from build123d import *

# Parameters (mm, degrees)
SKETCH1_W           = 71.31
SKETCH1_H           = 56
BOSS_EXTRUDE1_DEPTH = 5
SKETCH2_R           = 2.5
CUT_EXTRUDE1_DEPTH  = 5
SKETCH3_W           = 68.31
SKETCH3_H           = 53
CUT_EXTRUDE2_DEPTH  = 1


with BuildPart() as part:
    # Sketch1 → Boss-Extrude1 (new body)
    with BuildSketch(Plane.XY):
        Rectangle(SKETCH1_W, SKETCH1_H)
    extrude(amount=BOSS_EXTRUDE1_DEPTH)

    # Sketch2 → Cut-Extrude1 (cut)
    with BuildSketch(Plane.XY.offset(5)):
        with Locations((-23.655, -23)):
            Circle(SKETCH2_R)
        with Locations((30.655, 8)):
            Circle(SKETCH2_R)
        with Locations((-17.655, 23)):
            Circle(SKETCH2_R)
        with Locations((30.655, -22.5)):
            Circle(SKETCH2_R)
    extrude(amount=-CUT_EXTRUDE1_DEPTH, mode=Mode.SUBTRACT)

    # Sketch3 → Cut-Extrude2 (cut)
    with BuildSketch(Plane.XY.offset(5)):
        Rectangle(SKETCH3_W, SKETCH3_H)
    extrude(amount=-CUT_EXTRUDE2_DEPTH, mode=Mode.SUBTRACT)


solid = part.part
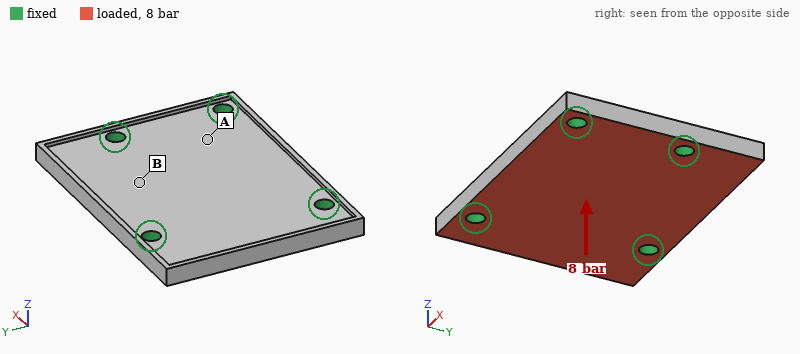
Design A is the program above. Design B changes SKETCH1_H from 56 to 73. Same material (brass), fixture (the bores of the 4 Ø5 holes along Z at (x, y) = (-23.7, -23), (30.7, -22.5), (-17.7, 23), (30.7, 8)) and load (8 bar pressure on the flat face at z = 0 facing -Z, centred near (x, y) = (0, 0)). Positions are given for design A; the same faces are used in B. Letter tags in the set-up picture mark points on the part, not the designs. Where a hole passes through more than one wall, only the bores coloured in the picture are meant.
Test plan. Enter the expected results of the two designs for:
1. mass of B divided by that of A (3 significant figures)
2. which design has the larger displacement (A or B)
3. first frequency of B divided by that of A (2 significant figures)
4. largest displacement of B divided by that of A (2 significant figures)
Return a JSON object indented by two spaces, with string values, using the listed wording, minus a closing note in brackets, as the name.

{
  "mass of B divided by that of A": "1.38",
  "which design has the larger displacement": "B",
  "first frequency of B divided by that of A": "0.69",
  "largest displacement of B divided by that of A": "2.0"
}
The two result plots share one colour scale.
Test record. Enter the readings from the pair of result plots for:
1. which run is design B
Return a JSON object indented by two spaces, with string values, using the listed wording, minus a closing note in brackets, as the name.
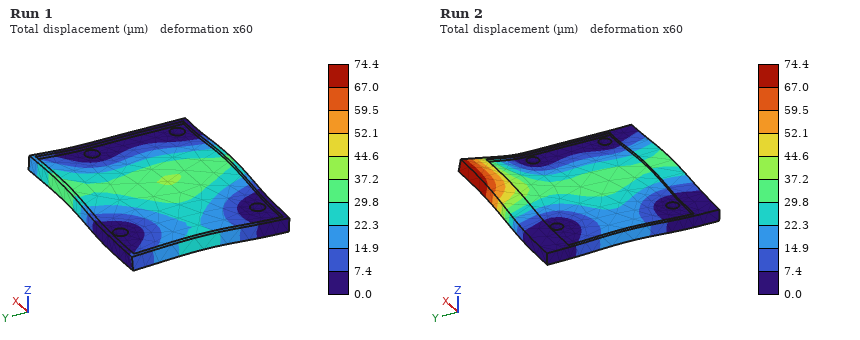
{
  "which run is design B": "Run 2"
}
